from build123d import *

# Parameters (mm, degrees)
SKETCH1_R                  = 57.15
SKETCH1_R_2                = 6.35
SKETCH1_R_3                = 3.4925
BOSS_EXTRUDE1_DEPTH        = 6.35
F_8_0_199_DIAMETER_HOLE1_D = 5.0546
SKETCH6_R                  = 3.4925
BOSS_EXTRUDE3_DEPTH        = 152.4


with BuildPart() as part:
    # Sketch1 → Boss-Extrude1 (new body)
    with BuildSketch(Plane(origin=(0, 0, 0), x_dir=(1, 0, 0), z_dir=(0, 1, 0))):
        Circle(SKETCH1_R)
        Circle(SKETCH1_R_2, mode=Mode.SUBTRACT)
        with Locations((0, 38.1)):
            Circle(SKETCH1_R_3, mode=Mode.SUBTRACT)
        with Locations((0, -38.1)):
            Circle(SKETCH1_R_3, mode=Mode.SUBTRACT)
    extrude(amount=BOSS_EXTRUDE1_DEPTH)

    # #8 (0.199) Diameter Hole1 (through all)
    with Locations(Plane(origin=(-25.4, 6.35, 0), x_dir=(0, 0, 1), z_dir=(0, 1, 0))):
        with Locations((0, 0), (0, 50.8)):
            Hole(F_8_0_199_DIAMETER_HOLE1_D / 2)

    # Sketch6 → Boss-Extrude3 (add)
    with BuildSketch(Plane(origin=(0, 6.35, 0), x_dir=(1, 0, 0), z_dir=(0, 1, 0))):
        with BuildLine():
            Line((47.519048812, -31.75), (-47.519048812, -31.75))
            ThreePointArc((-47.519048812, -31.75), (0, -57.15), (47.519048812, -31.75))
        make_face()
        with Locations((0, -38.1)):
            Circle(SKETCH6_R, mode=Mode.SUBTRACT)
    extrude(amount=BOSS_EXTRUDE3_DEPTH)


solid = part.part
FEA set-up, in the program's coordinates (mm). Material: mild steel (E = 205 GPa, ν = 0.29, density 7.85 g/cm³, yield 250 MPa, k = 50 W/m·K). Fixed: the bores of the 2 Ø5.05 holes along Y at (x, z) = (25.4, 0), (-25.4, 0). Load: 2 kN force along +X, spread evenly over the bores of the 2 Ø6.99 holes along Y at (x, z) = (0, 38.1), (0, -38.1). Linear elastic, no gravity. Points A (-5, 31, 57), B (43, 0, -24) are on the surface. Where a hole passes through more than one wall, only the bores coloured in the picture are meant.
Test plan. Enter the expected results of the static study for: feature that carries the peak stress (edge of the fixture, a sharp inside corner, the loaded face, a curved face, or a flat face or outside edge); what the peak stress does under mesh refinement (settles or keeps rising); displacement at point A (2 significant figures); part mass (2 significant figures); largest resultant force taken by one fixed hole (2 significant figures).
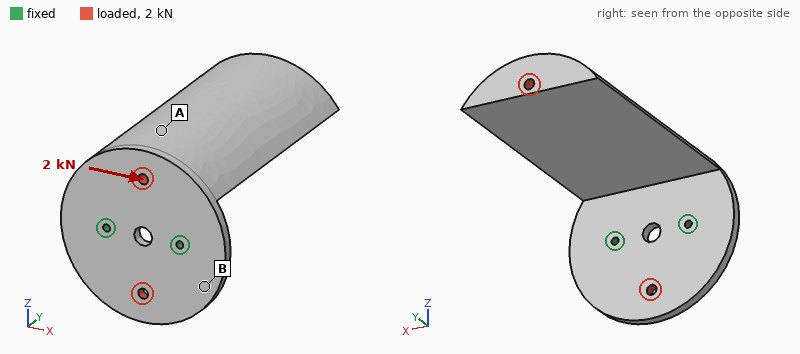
edge of the fixture
keeps rising
0.057 mm
2.5 kg
2.9 kN
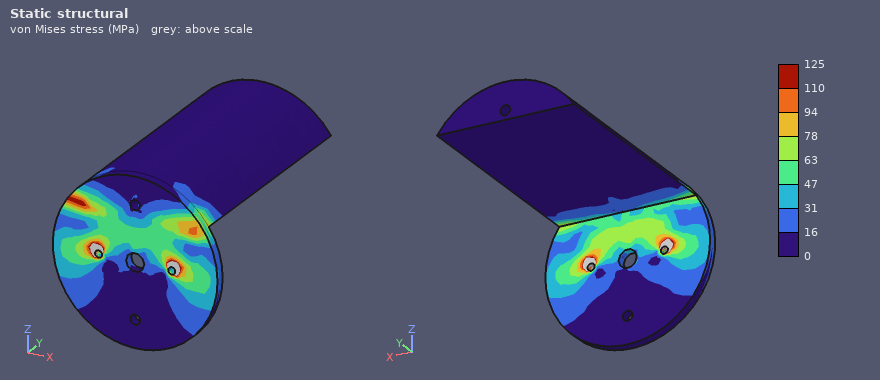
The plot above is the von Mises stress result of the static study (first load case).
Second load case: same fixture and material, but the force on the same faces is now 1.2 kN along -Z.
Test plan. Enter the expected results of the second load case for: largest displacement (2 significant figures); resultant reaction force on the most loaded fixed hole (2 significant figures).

1.3 mm
600 N
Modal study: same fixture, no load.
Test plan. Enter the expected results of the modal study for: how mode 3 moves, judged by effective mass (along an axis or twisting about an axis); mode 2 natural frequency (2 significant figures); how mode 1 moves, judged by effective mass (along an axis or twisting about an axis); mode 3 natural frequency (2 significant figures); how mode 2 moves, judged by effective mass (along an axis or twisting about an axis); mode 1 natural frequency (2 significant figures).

along Y
320 Hz
along Z
940 Hz
along X
130 Hz
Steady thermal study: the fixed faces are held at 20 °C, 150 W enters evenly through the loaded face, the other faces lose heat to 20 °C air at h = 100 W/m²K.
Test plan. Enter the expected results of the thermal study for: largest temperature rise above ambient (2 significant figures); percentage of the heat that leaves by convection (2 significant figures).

47 K
90 %
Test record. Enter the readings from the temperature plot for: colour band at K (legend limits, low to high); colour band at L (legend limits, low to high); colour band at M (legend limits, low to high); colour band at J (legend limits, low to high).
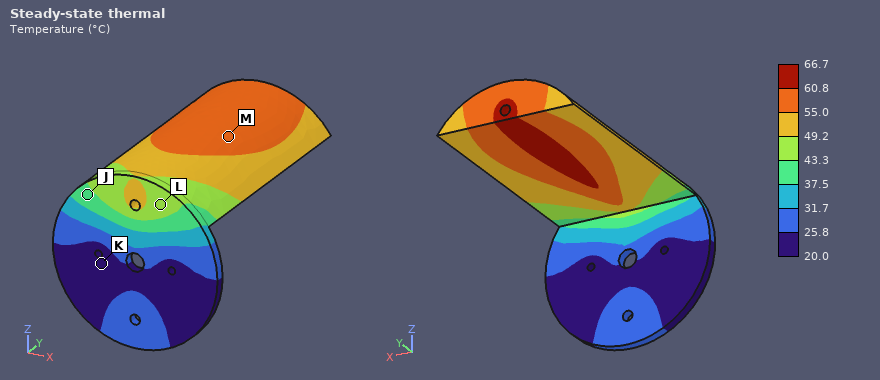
20.0 to 25.8 °C
43.3 to 49.2 °C
55.0 to 60.8 °C
37.5 to 43.3 °C
